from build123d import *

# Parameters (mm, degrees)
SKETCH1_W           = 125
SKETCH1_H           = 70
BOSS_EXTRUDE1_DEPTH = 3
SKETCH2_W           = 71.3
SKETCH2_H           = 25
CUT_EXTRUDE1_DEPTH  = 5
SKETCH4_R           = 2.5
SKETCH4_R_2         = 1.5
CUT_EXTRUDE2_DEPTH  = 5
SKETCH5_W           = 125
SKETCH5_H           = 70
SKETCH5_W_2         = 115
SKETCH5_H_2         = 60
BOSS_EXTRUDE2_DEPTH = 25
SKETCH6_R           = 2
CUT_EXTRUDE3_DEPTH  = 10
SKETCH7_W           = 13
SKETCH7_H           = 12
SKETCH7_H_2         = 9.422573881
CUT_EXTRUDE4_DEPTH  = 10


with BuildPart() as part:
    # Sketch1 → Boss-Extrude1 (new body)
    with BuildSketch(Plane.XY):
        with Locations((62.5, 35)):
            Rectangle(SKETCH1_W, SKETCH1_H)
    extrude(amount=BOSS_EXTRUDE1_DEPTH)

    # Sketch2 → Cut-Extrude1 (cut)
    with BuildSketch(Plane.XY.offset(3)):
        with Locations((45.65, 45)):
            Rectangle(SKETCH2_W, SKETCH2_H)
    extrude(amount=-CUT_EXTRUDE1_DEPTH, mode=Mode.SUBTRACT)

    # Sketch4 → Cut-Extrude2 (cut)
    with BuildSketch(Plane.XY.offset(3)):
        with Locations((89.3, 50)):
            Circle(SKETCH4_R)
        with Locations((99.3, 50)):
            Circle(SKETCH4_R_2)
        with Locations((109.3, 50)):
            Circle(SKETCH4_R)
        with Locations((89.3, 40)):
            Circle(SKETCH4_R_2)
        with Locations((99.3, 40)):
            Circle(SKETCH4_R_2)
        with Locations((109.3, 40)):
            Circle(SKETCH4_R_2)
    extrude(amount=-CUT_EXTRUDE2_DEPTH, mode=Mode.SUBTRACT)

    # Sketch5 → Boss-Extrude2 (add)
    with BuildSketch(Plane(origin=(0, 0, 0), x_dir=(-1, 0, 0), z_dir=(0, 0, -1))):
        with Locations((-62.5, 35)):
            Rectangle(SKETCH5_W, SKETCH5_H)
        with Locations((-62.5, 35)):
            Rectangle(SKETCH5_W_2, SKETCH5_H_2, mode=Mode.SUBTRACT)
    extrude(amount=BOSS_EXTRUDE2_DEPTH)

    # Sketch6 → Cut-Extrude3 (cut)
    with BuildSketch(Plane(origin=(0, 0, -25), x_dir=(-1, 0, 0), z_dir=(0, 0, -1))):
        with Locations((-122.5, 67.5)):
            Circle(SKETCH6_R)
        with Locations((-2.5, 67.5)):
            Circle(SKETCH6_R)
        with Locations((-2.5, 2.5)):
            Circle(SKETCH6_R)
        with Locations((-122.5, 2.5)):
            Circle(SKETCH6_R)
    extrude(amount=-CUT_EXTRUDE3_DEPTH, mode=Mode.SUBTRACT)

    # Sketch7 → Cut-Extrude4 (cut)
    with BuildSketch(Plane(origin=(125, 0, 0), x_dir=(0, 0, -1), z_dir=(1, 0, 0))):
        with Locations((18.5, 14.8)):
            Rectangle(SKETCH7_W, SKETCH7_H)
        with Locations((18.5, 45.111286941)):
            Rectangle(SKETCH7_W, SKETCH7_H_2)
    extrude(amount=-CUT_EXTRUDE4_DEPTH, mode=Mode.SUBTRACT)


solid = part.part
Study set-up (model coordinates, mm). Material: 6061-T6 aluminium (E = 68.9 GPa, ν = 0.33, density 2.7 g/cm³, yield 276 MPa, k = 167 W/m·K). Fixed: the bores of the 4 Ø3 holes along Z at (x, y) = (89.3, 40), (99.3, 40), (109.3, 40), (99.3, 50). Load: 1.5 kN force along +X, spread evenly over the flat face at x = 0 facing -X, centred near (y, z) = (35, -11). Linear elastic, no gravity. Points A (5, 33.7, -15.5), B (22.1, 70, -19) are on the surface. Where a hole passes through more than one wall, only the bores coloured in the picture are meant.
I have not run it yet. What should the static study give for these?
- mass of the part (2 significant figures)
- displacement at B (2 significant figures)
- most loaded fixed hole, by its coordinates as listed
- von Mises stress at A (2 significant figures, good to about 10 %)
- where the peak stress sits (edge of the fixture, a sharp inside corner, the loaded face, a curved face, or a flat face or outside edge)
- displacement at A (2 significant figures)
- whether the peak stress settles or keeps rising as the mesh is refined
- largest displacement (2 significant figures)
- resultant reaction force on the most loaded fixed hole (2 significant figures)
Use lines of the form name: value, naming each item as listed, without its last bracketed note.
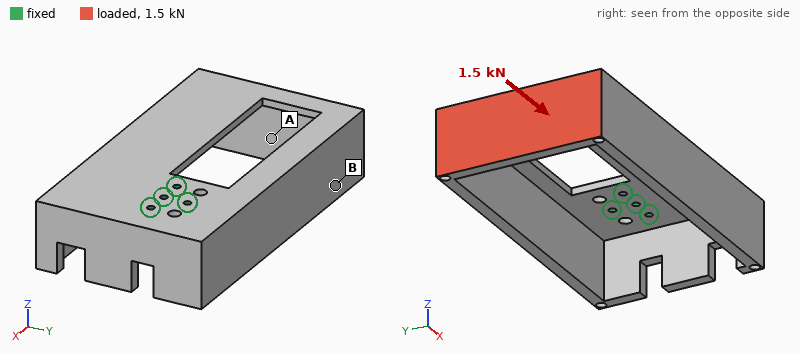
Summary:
mass of the part: 180 g
displacement at B: 0.57 mm
most loaded fixed hole, by its coordinates as listed: (109.3, 40)
von Mises stress at A: 21 MPa
where the peak stress sits: edge of the fixture
displacement at A: 0.79 mm
whether the peak stress settles or keeps rising as the mesh is refined: keeps rising
largest displacement: 0.93 mm
resultant reaction force on the most loaded fixed hole: 990 N
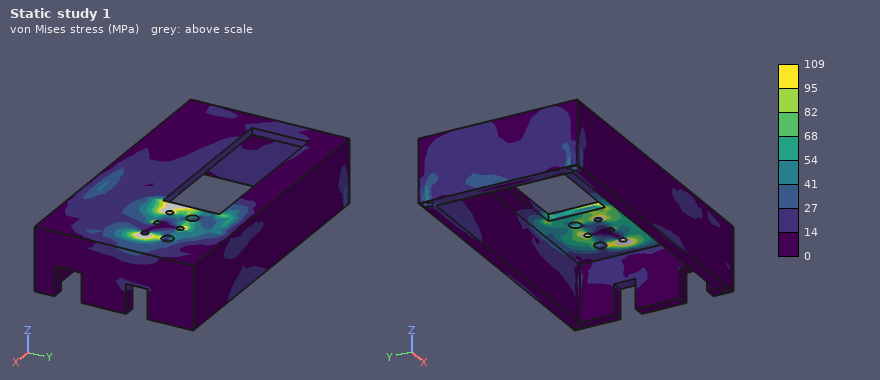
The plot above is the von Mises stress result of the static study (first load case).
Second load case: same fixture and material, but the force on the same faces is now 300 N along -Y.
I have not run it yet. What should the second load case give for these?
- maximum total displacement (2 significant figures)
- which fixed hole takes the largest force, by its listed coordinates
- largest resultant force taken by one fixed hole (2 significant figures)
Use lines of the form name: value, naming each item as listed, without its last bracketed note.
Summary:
maximum total displacement: 0.31 mm
which fixed hole takes the largest force, by its listed coordinates: (89.3, 40)
largest resultant force taken by one fixed hole: 1.2 kN
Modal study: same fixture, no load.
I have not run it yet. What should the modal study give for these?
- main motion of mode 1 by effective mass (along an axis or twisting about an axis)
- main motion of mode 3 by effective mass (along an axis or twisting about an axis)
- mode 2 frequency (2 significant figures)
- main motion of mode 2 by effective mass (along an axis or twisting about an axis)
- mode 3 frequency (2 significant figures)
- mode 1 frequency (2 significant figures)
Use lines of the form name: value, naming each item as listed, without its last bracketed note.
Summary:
main motion of mode 1 by effective mass: along Z
main motion of mode 3 by effective mass: along Y
mode 2 frequency: 590 Hz
main motion of mode 2 by effective mass: along Y
mode 3 frequency: 1200 Hz
mode 1 frequency: 290 Hz
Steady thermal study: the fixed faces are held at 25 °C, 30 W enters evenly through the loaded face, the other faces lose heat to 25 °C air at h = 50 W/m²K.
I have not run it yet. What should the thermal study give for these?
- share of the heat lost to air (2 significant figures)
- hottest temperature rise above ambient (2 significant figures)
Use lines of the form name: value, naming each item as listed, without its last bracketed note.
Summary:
share of the heat lost to air: 68 %
hottest temperature rise above ambient: 34 K
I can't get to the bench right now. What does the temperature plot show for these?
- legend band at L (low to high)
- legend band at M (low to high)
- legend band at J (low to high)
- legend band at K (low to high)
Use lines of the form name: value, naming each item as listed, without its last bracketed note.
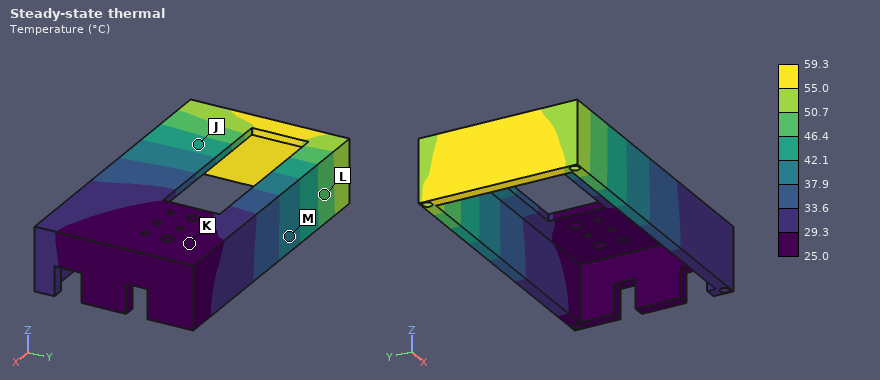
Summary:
legend band at L: 46.4 to 50.7 °C
legend band at M: 37.9 to 42.1 °C
legend band at J: 42.1 to 46.4 °C
legend band at K: 25.0 to 29.3 °C
